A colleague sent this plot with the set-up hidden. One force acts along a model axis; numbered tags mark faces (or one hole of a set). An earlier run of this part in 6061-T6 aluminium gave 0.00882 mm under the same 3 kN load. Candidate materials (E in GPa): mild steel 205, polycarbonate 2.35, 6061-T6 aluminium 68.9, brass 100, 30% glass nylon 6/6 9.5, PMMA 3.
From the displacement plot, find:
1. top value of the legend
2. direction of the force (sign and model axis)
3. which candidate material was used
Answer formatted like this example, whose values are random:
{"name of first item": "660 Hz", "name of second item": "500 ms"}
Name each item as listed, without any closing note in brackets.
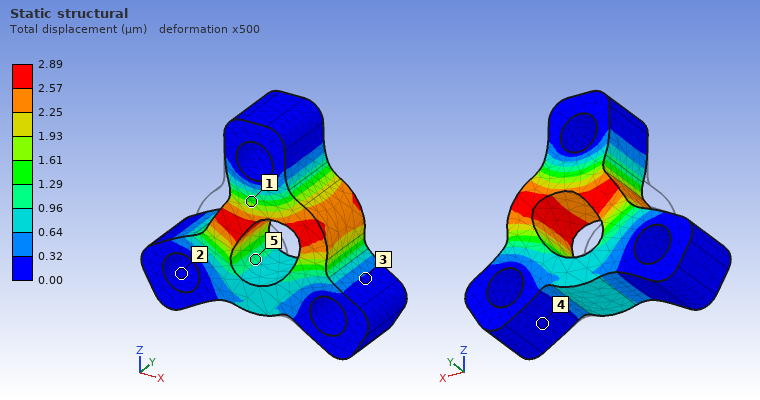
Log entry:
{"top value of the legend": "2.89 µm", "direction of the force": "+X", "which candidate material was used": "mild steel"}
